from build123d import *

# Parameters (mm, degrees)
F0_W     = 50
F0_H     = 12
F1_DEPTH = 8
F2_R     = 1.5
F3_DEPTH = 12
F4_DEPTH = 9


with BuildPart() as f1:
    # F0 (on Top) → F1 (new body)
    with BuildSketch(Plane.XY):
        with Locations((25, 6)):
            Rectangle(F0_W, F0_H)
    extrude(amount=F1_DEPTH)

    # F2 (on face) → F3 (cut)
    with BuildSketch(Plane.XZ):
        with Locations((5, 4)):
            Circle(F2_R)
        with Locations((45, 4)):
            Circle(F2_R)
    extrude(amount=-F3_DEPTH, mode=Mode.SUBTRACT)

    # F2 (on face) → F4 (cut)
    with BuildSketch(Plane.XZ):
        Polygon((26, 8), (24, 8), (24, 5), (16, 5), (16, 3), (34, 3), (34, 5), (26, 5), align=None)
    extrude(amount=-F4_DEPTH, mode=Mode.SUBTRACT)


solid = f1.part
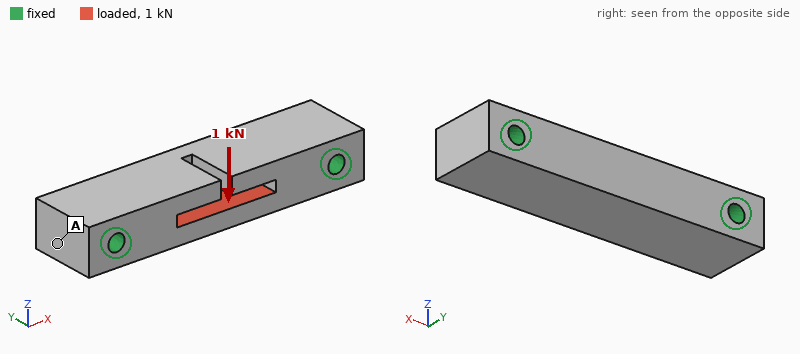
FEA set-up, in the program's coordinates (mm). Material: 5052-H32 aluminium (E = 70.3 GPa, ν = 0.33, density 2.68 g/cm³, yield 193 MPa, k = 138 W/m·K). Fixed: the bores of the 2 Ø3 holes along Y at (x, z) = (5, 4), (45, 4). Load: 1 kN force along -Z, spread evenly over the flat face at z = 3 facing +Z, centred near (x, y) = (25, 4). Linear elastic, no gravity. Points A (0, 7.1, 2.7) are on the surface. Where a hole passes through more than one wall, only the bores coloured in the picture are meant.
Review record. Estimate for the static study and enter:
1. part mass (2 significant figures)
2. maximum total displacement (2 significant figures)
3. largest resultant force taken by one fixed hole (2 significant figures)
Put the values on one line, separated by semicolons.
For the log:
11 g; 34 µm; 580 N
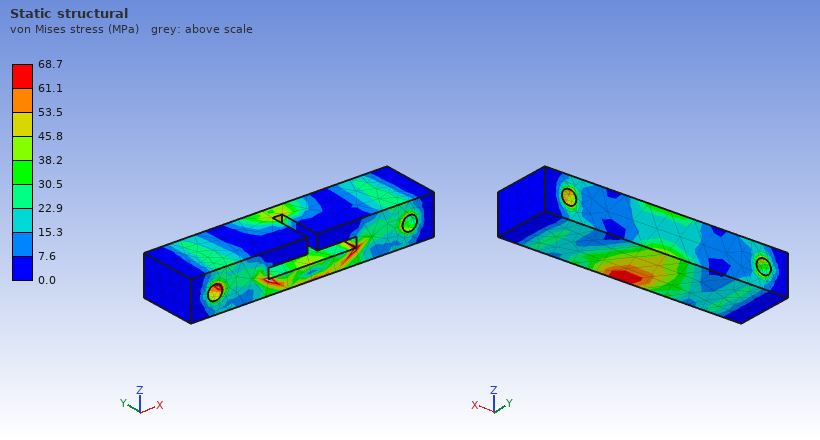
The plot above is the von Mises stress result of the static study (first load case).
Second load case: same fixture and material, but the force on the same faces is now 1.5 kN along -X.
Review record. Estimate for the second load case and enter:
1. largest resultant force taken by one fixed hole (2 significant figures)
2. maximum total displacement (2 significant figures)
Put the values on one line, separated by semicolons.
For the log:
750 N; 5.4 µm
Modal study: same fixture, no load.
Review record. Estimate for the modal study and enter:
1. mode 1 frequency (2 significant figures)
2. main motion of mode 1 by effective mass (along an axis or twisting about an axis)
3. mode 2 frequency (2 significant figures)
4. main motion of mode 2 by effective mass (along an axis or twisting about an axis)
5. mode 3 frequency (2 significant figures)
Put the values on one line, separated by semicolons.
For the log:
18 kHz; along Z; 28 kHz; along Y; 32 kHz
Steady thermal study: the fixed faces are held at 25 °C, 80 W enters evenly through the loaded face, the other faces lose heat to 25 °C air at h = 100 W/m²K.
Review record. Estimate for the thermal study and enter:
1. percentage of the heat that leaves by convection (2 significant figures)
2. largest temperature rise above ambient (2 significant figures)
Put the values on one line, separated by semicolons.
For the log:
6.0 %; 74 K
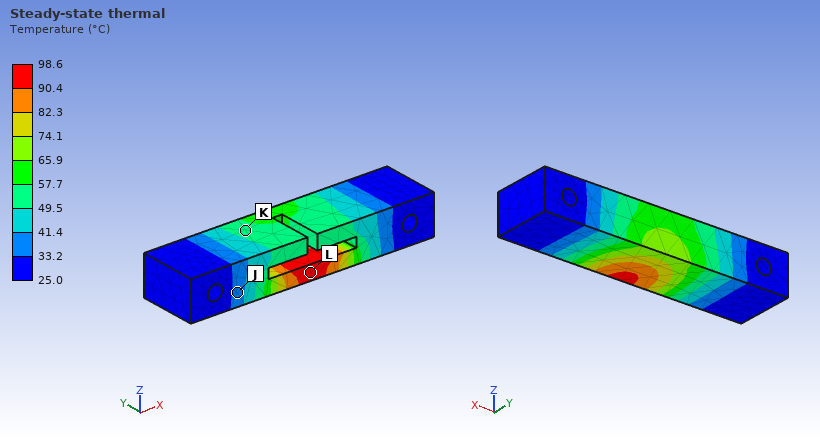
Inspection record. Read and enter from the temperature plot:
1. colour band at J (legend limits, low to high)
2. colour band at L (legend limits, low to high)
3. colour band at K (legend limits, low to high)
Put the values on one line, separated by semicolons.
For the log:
33.2 to 41.4 °C; 90.4 to 98.6 °C; 49.5 to 57.7 °C
